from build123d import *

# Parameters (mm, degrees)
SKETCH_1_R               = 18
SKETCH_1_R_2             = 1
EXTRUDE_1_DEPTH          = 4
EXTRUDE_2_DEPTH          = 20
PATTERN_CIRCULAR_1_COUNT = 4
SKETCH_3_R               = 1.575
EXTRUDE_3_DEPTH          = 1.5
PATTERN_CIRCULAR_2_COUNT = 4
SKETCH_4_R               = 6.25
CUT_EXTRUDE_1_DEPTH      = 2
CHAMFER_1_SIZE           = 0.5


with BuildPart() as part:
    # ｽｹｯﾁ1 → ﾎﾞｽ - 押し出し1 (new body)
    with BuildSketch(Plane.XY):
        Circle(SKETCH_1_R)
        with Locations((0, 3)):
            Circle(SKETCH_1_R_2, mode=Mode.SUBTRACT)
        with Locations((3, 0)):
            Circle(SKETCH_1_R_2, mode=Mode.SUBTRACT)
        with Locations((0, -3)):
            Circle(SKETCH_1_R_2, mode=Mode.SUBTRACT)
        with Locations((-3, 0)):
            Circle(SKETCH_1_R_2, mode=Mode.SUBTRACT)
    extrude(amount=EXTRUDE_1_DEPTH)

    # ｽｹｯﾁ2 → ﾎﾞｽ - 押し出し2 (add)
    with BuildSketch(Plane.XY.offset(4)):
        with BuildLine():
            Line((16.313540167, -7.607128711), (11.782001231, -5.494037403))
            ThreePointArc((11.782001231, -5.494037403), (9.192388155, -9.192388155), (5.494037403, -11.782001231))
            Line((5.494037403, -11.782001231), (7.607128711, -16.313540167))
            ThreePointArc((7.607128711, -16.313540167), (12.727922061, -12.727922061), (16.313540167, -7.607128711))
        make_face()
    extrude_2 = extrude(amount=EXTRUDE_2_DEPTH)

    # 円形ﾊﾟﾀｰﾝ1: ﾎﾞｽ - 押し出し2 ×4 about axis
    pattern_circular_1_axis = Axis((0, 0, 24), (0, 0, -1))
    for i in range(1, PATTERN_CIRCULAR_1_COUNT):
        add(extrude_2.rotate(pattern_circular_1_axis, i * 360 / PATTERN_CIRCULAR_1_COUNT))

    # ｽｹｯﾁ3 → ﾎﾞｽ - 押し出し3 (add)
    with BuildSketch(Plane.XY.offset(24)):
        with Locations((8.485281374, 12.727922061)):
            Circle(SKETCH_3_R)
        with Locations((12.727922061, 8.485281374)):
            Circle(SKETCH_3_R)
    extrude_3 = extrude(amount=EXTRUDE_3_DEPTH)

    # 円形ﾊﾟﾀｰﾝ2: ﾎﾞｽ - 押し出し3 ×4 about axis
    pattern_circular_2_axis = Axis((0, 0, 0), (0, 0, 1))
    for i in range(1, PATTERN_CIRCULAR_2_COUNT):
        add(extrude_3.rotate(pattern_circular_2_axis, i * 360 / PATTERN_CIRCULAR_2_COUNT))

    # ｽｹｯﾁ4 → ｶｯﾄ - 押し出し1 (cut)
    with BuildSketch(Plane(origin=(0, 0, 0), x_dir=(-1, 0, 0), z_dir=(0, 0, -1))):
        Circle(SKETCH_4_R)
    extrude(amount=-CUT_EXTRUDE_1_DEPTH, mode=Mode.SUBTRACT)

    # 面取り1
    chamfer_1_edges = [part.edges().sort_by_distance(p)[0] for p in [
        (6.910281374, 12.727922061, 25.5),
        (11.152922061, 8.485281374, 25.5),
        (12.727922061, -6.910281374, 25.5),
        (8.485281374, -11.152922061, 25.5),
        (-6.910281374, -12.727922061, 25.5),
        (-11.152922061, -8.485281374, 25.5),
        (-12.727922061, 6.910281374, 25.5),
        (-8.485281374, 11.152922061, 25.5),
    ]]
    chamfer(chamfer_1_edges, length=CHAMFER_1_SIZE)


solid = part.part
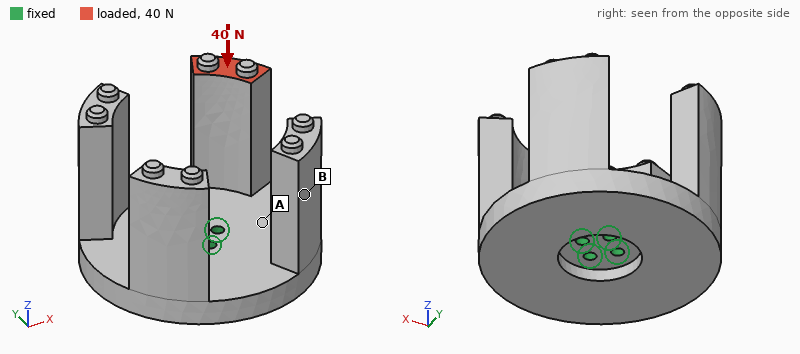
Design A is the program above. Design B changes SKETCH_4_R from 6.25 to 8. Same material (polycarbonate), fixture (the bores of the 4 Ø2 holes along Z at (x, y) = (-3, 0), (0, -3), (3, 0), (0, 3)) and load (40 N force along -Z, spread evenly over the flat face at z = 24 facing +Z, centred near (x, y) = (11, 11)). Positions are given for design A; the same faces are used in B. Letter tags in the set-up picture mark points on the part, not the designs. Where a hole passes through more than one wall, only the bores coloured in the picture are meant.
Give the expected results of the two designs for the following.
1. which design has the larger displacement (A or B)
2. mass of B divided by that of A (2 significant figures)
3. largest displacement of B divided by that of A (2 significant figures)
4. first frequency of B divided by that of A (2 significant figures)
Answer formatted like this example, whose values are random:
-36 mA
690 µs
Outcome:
B
0.98
1.2
0.92
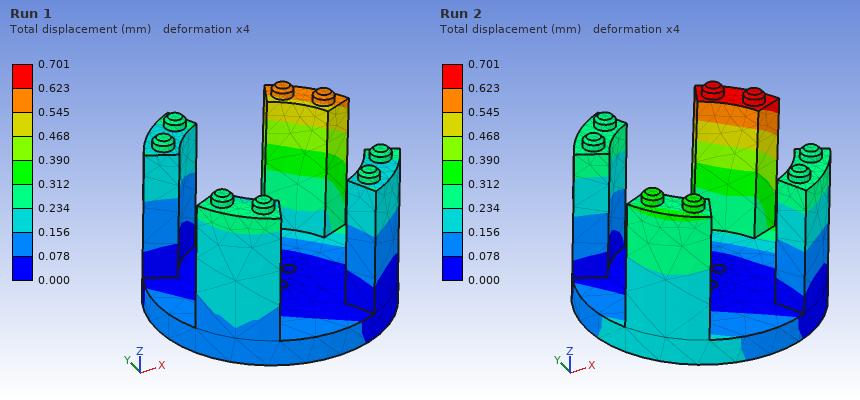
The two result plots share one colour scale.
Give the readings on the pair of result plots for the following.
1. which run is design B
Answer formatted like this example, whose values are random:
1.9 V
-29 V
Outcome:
Run 2
